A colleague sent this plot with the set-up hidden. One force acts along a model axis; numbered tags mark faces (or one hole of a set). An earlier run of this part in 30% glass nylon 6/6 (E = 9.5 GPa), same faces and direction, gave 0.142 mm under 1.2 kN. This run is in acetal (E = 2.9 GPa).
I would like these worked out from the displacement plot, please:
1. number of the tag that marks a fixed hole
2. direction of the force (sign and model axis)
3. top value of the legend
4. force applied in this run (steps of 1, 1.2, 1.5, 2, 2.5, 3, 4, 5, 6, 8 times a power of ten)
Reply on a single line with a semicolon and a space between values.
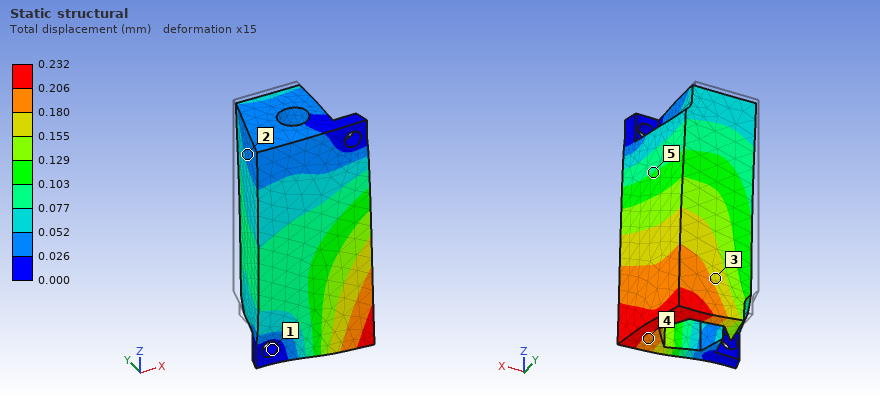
1; -Y; 0.232 mm; 600 N
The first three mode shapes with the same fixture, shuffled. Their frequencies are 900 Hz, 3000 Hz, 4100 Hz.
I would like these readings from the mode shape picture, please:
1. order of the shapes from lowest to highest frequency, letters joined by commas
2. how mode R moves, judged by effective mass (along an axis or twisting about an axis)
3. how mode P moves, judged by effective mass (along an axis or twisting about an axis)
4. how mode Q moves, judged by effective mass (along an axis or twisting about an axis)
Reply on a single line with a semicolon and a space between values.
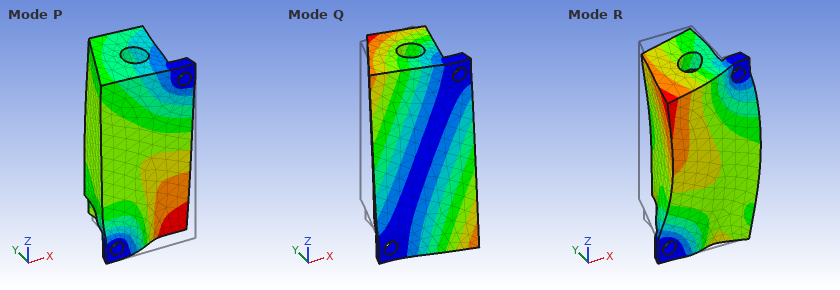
Q, P, R; along X; along Y; along X
